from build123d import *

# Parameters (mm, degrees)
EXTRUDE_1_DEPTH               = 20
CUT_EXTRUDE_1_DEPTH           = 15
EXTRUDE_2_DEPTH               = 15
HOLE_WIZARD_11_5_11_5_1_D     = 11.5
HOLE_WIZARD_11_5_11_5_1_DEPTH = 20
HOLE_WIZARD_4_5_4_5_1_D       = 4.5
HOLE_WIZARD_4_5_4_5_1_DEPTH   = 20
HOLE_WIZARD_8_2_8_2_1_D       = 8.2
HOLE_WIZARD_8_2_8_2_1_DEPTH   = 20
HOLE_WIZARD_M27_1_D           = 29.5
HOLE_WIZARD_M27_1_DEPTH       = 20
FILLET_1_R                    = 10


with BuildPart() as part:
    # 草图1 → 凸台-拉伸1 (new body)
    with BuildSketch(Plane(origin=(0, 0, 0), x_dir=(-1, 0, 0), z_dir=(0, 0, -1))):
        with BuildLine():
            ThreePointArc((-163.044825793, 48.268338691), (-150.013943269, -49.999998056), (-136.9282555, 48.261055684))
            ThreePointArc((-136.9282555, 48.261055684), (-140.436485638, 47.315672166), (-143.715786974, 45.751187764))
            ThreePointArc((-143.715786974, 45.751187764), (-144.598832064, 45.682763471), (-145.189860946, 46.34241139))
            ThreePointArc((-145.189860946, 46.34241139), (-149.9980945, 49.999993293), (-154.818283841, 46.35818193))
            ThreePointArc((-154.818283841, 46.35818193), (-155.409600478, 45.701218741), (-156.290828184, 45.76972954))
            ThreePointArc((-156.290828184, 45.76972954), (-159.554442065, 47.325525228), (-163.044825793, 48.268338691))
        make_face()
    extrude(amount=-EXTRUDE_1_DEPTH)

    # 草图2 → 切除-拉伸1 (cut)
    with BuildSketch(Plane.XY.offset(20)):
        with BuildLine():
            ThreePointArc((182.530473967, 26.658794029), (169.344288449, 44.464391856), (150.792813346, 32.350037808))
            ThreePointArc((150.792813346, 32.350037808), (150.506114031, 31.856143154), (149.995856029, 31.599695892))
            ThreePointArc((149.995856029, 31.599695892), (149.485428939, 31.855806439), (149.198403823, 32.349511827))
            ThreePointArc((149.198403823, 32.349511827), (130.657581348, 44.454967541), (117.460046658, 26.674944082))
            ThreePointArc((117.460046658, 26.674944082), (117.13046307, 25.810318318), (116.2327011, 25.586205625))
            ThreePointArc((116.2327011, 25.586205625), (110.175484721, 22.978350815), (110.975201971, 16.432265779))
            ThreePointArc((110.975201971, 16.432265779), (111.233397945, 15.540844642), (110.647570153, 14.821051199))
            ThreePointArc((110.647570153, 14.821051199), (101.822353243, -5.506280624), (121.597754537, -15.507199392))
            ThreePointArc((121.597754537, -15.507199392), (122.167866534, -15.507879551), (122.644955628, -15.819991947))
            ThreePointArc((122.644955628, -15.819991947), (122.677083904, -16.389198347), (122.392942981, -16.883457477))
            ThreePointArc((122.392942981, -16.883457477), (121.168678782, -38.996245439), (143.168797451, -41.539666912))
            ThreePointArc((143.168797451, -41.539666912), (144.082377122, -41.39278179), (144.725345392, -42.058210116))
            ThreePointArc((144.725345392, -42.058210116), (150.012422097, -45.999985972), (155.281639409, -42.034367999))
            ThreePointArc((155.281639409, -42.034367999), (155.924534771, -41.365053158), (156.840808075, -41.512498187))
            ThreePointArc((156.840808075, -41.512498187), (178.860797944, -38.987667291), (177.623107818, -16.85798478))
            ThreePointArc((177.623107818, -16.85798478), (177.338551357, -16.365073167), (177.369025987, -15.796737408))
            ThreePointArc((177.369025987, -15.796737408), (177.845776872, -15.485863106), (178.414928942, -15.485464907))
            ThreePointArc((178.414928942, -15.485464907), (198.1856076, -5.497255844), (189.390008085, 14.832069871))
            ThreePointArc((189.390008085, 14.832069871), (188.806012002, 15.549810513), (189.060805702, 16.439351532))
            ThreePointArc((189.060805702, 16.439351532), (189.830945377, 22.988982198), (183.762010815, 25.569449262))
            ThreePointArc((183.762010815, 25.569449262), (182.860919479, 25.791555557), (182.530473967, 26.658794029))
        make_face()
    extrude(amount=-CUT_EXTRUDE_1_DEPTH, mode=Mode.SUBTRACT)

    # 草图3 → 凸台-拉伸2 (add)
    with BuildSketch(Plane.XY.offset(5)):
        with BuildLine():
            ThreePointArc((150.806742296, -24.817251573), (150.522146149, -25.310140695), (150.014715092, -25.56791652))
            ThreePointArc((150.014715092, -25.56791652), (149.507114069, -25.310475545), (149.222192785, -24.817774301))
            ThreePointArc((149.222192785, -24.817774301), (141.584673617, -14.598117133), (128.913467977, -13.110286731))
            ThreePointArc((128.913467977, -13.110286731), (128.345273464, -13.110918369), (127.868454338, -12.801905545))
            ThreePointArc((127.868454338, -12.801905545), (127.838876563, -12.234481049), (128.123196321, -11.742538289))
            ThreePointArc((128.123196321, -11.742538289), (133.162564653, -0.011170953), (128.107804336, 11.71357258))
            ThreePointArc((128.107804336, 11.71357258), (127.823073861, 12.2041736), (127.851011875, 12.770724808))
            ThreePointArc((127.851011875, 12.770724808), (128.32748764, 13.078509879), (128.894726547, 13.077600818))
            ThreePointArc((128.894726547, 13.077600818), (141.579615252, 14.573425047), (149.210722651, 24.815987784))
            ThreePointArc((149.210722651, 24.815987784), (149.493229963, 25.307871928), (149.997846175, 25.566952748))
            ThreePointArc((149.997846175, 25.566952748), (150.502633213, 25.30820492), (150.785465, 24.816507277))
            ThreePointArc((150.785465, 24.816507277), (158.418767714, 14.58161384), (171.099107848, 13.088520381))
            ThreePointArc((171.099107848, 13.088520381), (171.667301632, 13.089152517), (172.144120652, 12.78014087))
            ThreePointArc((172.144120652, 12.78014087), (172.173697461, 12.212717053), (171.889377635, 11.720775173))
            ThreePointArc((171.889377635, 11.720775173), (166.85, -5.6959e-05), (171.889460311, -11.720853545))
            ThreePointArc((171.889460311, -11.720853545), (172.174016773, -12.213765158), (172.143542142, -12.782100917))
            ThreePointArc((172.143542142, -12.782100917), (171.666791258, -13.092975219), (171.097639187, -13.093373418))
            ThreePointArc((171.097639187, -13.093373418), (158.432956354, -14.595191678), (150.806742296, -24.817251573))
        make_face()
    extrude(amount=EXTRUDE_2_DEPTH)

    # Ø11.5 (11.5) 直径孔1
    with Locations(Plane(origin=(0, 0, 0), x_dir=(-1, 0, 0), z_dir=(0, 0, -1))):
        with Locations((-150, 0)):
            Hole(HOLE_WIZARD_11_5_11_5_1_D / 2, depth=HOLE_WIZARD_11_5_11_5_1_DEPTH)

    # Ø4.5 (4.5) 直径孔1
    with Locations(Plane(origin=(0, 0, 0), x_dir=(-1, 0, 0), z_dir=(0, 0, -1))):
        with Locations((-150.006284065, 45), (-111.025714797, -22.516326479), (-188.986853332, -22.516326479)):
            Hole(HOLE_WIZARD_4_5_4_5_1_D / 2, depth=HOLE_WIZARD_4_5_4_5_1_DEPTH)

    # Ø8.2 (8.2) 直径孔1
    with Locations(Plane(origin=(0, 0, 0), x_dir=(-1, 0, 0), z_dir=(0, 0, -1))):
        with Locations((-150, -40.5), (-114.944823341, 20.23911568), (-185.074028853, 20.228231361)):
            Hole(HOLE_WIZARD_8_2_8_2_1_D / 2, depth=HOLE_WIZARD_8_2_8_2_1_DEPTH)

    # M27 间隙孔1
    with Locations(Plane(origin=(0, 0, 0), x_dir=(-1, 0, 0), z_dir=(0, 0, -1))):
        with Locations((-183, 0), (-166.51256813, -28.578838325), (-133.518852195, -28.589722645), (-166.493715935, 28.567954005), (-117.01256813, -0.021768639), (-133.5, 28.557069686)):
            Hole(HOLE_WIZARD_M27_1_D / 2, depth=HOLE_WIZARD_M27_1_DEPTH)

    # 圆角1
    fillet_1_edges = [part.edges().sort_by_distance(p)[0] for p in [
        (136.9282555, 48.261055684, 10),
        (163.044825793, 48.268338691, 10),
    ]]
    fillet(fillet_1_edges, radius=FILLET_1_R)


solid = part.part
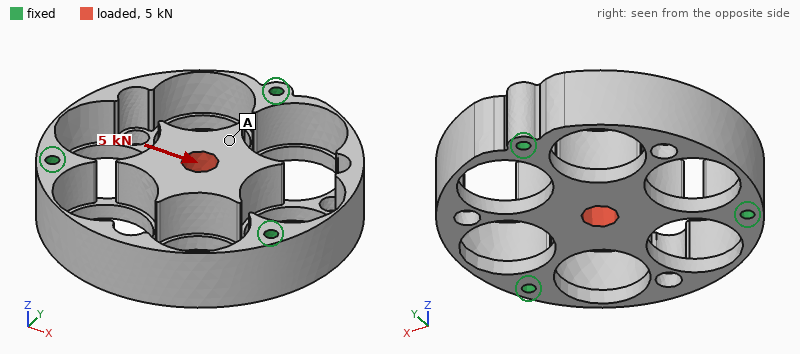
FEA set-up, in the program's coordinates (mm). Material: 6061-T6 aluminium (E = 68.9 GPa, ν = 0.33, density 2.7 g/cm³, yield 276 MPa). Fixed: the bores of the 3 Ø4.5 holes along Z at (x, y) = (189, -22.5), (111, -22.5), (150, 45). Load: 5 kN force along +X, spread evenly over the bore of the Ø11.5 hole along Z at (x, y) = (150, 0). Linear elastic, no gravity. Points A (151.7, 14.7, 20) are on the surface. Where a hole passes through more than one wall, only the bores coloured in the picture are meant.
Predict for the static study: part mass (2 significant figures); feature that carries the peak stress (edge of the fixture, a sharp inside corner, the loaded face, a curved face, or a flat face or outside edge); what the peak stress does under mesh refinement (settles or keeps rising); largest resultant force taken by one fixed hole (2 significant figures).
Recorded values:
140 g
a sharp inside corner
keeps rising
2.4 kN
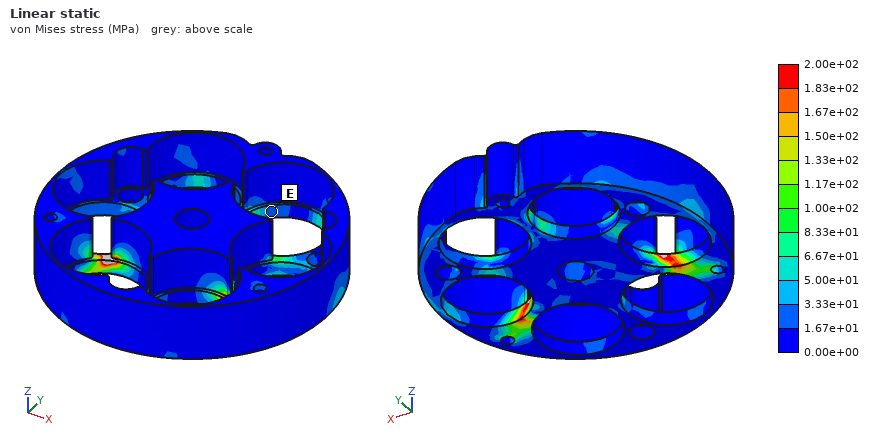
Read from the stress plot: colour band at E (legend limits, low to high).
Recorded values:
1.67e+01 to 3.33e+01 MPa
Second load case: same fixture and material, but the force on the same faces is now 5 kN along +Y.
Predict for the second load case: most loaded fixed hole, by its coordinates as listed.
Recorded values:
(150, 45)
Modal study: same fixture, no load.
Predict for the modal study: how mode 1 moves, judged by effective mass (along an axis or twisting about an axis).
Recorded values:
along Z
